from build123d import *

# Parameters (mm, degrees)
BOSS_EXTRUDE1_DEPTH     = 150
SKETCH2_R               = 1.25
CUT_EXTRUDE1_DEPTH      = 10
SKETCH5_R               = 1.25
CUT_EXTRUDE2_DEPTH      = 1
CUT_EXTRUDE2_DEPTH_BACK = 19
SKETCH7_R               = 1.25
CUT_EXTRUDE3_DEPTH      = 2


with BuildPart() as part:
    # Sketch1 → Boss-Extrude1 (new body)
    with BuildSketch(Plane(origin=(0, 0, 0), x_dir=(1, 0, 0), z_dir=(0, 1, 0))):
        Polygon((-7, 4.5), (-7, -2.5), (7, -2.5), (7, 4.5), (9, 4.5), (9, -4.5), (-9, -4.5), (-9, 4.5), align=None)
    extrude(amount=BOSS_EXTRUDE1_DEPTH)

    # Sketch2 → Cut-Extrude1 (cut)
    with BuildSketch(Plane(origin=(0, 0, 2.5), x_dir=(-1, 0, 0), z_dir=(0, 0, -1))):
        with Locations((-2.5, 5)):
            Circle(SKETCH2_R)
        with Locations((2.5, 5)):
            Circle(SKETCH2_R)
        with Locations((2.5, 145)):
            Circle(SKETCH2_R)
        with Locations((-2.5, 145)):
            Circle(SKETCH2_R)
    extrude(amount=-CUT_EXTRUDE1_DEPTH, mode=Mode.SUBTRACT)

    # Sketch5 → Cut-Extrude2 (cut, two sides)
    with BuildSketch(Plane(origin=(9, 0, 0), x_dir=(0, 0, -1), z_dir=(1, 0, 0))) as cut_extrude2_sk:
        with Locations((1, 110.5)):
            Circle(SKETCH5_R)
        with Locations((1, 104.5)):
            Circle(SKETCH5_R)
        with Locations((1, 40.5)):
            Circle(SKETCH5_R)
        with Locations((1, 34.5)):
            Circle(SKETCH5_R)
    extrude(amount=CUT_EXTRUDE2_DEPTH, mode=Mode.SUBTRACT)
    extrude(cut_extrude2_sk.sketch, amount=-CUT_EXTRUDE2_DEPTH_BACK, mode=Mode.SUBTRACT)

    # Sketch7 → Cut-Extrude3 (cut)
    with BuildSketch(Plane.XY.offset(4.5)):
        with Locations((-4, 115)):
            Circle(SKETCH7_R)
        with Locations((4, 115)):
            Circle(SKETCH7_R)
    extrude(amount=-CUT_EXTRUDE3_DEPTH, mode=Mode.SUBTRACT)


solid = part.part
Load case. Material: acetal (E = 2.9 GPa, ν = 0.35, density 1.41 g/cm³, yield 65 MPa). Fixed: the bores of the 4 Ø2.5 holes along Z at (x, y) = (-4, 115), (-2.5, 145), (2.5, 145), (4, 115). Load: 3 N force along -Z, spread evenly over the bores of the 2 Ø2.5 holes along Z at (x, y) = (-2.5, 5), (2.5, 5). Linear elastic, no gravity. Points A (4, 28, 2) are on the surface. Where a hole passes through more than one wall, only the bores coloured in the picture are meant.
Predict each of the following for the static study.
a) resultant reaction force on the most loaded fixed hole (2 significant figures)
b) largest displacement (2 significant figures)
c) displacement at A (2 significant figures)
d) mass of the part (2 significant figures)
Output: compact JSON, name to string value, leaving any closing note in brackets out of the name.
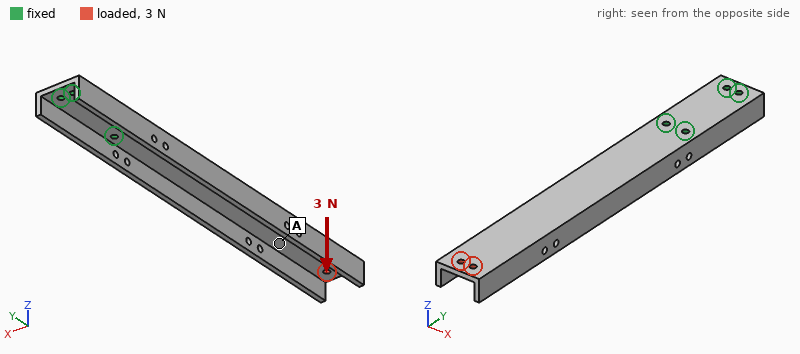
{"resultant reaction force on the most loaded fixed hole": "12 N", "largest displacement": "1.4 mm", "displacement at A": "0.94 mm", "mass of the part": "13 g"}
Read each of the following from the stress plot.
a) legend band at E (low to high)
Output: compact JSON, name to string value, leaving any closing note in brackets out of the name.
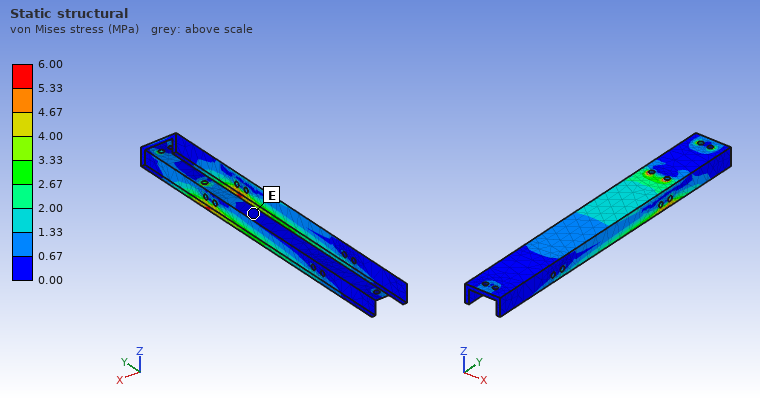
{"legend band at E": "0.00 to 0.67 MPa"}
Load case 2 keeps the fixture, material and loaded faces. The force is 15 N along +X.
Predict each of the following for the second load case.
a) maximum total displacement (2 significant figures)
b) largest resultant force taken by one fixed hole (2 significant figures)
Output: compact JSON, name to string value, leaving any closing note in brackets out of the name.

{"maximum total displacement": "1.6 mm", "largest resultant force taken by one fixed hole": "98 N"}
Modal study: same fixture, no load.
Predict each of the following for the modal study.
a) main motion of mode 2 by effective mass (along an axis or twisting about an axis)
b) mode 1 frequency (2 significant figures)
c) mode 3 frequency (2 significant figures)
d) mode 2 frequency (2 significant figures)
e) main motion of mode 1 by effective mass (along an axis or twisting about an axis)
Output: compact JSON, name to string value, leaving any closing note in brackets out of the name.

{"main motion of mode 2 by effective mass": "along X", "mode 1 frequency": "140 Hz", "mode 3 frequency": "440 Hz", "mode 2 frequency": "270 Hz", "main motion of mode 1 by effective mass": "along Z"}
